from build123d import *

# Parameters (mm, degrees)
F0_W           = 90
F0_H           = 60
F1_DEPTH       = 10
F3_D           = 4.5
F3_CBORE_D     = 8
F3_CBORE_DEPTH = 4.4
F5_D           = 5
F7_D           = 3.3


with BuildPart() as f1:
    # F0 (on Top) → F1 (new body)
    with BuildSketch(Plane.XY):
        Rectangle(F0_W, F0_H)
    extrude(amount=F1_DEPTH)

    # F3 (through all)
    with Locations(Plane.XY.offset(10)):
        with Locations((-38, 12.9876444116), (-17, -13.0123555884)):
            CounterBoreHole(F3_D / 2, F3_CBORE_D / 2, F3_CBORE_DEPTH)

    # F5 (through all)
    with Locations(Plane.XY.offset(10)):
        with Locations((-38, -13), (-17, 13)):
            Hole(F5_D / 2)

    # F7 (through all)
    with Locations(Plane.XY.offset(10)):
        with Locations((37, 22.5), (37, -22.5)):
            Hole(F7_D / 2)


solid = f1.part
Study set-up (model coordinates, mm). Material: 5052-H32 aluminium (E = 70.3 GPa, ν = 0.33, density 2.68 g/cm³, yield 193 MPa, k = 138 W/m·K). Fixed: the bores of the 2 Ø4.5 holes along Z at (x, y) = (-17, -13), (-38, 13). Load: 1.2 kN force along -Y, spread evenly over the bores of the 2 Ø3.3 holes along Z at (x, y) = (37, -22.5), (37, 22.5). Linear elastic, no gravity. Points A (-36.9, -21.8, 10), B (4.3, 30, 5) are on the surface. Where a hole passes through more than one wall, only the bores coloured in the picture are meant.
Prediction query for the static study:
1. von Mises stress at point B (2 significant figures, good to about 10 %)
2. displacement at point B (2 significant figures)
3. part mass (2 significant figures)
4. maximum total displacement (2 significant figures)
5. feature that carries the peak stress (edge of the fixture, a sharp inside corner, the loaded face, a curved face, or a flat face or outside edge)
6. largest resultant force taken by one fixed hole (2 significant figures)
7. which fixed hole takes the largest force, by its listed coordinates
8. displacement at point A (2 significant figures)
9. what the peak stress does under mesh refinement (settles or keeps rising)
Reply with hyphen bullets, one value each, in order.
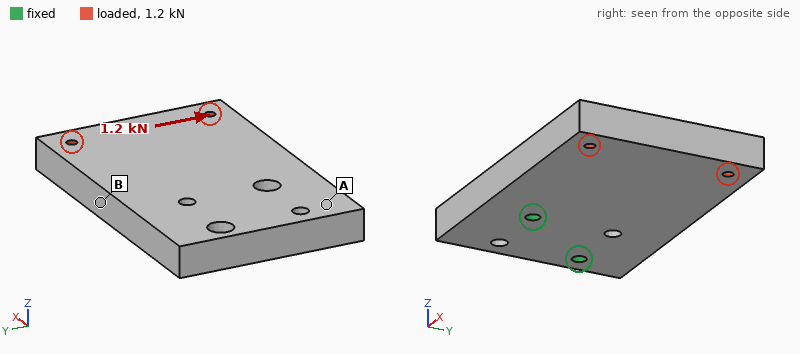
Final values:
- 7.9 MPa
- 16 µm
- 140 g
- 33 µm
- edge of the fixture
- 2.6 kN
- (-17, -13)
- 6.0 µm
- keeps rising
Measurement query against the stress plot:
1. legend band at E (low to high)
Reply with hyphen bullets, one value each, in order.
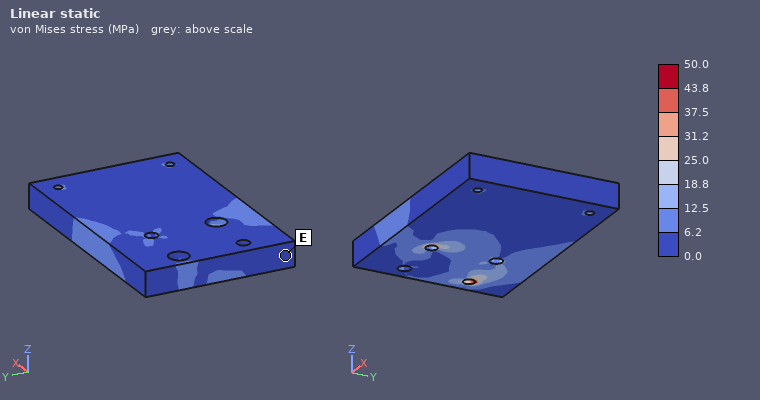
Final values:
- 0.0 to 6.2 MPa
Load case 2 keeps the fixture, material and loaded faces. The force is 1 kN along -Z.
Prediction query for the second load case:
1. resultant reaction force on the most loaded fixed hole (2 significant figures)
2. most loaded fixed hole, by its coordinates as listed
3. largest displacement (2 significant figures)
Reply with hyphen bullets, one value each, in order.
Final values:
- 1.6 kN
- (-17, -13)
- 0.48 mm
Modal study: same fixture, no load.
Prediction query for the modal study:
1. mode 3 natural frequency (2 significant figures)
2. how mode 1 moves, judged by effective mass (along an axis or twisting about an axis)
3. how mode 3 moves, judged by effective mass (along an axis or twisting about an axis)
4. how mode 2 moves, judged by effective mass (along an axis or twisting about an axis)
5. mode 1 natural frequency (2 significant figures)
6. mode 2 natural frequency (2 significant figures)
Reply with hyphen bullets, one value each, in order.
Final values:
- 5000 Hz
- along Z
- along Y
- twisting about X
- 1300 Hz
- 3500 Hz
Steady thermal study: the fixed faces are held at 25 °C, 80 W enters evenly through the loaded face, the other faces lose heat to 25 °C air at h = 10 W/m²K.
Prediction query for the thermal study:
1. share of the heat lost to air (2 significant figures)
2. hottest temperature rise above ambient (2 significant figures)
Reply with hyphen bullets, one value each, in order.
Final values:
- 5.6 %
- 74 K
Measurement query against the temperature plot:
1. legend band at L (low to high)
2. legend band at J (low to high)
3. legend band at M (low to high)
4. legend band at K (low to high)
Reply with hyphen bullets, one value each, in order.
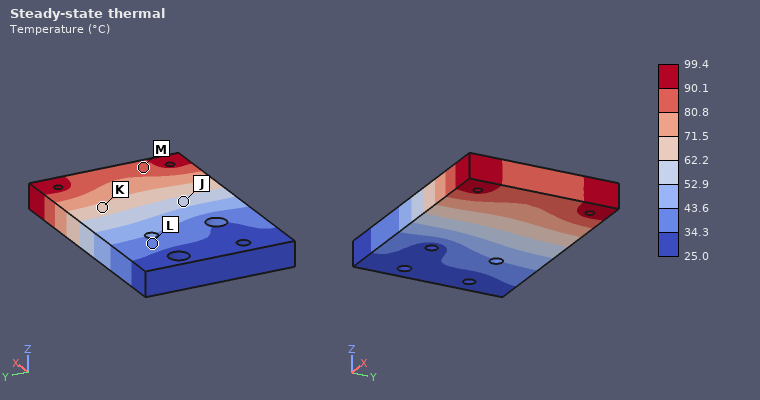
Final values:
- 34.3 to 43.6 °C
- 52.9 to 62.2 °C
- 80.8 to 90.1 °C
- 62.2 to 71.5 °C
